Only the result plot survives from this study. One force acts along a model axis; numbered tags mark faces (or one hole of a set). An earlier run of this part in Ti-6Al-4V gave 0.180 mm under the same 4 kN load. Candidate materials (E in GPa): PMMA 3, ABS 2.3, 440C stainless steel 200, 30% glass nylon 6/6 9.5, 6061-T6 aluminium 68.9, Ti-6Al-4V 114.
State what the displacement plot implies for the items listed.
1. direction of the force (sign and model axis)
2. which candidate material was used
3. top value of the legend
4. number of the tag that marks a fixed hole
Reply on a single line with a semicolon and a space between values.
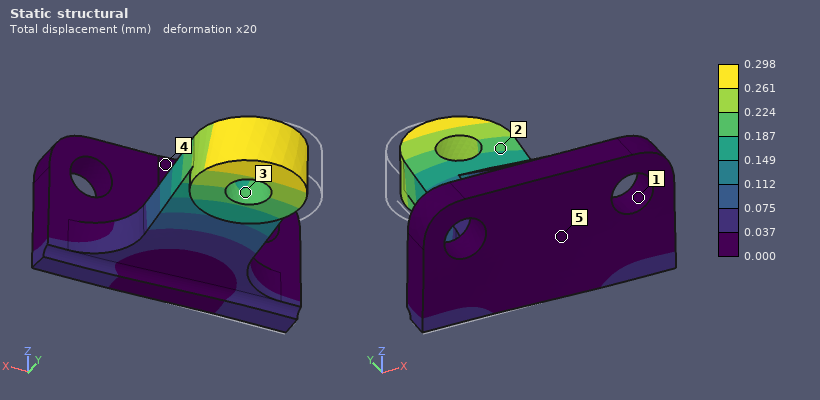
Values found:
+X; 6061-T6 aluminium; 0.298 mm; 1
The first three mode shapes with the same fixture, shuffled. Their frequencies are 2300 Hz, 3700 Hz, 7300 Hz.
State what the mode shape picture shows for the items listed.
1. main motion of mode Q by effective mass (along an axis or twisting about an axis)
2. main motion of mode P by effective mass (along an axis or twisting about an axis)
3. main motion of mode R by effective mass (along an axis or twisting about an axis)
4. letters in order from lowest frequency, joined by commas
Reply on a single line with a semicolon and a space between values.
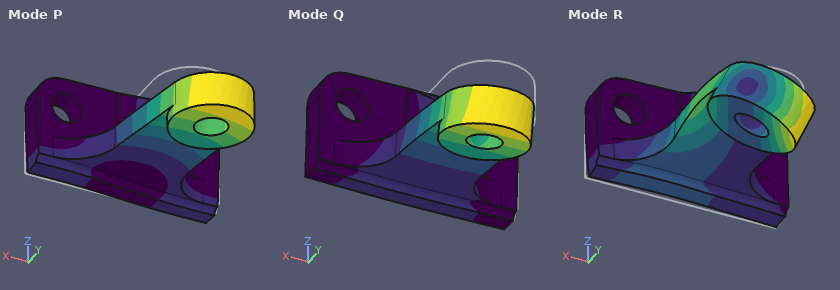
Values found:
along Z; along X; along Y; Q, P, R
